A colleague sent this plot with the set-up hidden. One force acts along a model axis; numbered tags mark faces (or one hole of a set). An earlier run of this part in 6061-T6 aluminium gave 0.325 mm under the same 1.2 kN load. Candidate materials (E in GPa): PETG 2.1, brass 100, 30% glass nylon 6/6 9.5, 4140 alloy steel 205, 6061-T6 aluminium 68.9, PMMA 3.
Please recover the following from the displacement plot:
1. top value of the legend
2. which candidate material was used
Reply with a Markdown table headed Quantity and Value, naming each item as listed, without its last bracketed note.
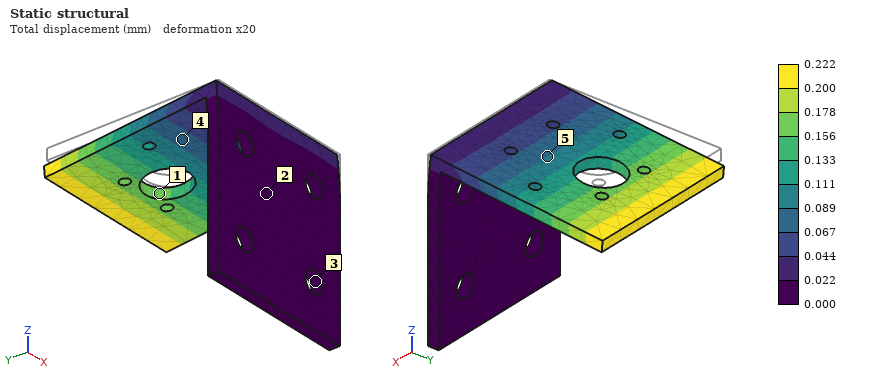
| Quantity | Value |
|---|---|
| top value of the legend | 0.222 mm |
| which candidate material was used | brass |
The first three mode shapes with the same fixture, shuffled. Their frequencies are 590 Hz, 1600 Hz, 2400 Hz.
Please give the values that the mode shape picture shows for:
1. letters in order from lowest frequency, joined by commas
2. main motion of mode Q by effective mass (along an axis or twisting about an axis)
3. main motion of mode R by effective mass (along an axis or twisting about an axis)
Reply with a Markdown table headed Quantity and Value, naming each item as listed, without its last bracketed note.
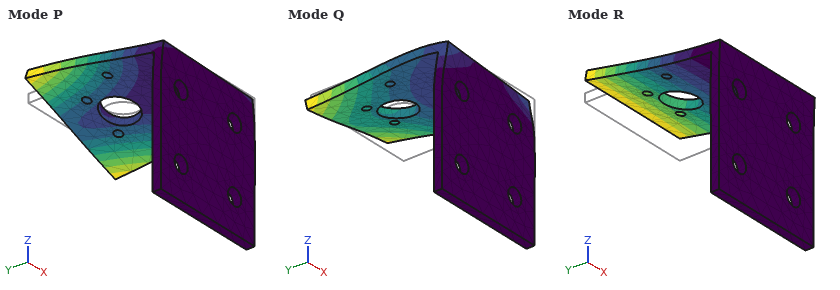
| Quantity | Value |
|---|---|
| letters in order from lowest frequency, joined by commas | R, P, Q |
| main motion of mode Q by effective mass | along X |
| main motion of mode R by effective mass | along Z |
